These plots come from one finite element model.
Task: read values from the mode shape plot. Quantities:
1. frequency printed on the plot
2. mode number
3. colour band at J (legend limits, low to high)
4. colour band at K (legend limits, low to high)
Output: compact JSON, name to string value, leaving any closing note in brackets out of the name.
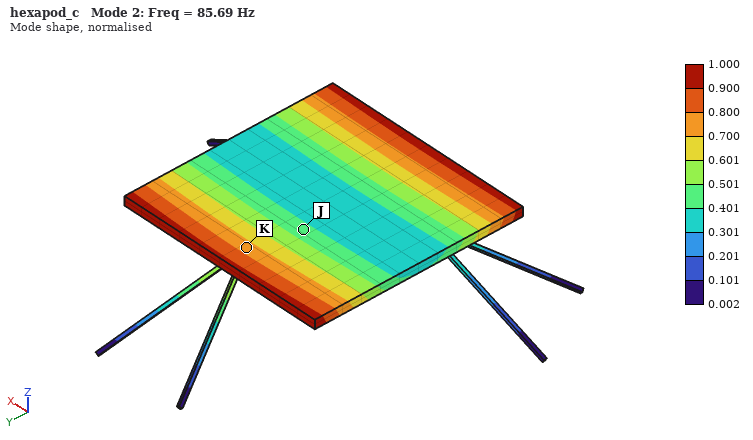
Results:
{"frequency printed on the plot": "85.69 Hz", "mode number": "2", "colour band at J": "0.401 to 0.501", "colour band at K": "0.700 to 0.800"}
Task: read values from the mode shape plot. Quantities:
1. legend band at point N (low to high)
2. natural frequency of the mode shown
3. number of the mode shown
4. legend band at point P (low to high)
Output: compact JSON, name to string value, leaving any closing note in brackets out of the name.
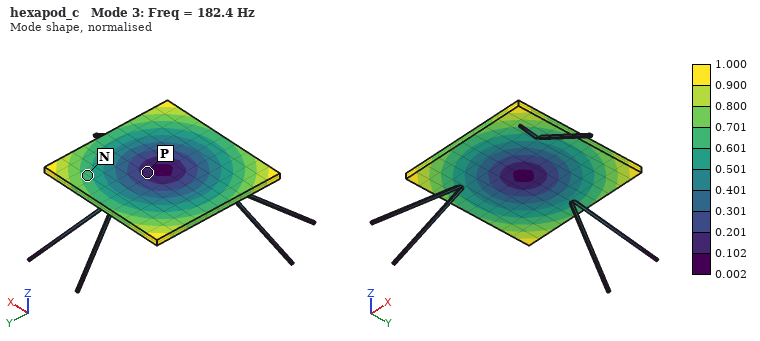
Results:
{"legend band at point N": "0.601 to 0.701", "natural frequency of the mode shown": "182.4 Hz", "number of the mode shown": "3", "legend band at point P": "0.102 to 0.201"}
